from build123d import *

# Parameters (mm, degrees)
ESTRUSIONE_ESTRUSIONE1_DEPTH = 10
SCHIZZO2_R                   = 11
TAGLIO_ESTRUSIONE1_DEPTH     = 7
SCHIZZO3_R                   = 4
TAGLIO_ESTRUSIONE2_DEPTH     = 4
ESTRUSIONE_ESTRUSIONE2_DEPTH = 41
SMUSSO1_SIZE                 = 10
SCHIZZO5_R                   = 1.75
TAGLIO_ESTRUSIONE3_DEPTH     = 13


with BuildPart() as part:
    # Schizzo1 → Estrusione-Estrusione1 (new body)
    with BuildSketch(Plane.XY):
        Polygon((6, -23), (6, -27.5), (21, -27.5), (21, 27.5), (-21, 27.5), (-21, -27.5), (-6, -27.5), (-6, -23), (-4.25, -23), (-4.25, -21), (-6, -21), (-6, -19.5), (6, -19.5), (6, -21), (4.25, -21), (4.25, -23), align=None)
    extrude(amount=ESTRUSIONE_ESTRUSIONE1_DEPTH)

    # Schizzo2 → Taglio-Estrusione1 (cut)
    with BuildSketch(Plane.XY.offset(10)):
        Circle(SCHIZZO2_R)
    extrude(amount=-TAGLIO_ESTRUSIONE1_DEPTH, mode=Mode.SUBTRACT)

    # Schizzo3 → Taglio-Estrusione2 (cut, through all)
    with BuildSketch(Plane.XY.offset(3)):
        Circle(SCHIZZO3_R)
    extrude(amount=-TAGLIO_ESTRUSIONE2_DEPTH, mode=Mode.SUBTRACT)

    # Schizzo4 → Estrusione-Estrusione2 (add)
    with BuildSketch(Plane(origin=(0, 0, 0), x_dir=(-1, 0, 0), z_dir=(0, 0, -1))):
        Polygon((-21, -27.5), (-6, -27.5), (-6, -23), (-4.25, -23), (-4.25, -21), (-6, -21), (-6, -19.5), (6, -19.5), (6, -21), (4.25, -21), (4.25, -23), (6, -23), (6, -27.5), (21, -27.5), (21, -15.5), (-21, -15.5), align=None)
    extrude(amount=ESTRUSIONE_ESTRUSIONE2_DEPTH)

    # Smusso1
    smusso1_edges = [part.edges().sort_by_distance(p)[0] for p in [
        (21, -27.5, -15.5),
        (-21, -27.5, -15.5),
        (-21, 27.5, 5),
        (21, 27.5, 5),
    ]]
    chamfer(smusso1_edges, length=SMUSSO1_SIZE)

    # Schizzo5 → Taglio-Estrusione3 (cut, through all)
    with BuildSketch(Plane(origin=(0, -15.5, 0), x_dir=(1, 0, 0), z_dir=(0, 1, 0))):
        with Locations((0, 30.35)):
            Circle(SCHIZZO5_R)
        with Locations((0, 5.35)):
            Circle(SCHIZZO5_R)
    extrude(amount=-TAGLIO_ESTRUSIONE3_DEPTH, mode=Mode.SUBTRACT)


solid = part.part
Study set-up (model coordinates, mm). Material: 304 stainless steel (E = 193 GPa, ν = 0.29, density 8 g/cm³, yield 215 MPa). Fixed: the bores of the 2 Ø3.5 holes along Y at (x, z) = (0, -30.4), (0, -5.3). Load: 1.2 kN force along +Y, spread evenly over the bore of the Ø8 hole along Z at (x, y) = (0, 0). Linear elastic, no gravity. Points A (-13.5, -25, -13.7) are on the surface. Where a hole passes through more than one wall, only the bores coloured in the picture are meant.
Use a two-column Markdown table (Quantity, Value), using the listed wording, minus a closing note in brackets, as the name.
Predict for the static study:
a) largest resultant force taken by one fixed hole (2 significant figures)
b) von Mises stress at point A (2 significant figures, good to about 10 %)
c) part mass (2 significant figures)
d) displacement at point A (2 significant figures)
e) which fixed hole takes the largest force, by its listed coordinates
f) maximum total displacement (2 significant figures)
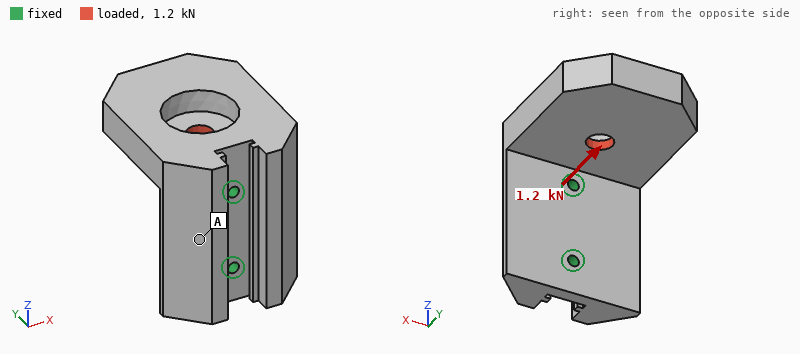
| Quantity | Value |
|---|---|
| largest resultant force taken by one fixed hole | 1.4 kN |
| von Mises stress at point A | 7.6 MPa |
| part mass | 240 g |
| displacement at point A | 2.0 µm |
| which fixed hole takes the largest force, by its listed coordinates | (0, -5.3) |
| maximum total displacement | 12 µm |
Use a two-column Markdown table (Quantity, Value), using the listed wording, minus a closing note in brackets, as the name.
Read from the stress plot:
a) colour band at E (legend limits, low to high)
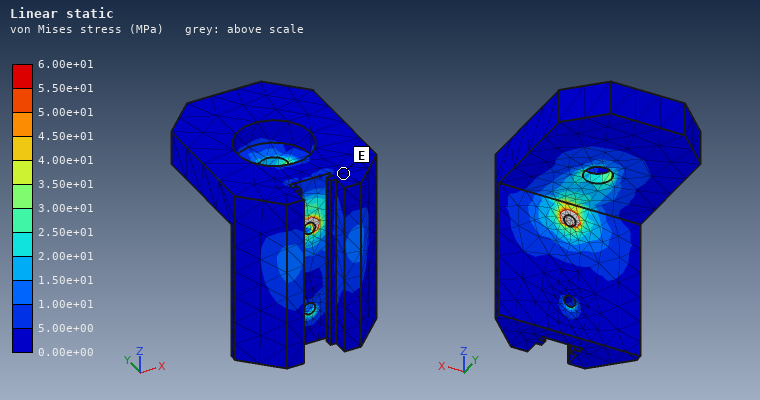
| Quantity | Value |
|---|---|
| colour band at E | 0.00e+00 to 5.00e+00 MPa |
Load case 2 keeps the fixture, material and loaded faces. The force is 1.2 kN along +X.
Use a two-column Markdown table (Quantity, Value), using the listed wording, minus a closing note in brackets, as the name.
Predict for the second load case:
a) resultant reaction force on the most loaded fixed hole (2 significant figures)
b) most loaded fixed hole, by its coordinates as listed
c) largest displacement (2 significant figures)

| Quantity | Value |
|---|---|
| resultant reaction force on the most loaded fixed hole | 1.5 kN |
| most loaded fixed hole, by its coordinates as listed | (0, -5.3) |
| largest displacement | 97 µm |
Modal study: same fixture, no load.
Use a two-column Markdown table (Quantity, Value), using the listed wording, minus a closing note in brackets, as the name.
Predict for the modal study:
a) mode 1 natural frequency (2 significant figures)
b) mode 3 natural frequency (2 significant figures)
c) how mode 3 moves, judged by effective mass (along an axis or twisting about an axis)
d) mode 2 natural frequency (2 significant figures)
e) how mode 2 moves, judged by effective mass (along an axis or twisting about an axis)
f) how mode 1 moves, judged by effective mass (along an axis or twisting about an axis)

| Quantity | Value |
|---|---|
| mode 1 natural frequency | 1500 Hz |
| mode 3 natural frequency | 6300 Hz |
| how mode 3 moves, judged by effective mass | twisting about Y |
| mode 2 natural frequency | 2000 Hz |
| how mode 2 moves, judged by effective mass | along Z |
| how mode 1 moves, judged by effective mass | along X |
